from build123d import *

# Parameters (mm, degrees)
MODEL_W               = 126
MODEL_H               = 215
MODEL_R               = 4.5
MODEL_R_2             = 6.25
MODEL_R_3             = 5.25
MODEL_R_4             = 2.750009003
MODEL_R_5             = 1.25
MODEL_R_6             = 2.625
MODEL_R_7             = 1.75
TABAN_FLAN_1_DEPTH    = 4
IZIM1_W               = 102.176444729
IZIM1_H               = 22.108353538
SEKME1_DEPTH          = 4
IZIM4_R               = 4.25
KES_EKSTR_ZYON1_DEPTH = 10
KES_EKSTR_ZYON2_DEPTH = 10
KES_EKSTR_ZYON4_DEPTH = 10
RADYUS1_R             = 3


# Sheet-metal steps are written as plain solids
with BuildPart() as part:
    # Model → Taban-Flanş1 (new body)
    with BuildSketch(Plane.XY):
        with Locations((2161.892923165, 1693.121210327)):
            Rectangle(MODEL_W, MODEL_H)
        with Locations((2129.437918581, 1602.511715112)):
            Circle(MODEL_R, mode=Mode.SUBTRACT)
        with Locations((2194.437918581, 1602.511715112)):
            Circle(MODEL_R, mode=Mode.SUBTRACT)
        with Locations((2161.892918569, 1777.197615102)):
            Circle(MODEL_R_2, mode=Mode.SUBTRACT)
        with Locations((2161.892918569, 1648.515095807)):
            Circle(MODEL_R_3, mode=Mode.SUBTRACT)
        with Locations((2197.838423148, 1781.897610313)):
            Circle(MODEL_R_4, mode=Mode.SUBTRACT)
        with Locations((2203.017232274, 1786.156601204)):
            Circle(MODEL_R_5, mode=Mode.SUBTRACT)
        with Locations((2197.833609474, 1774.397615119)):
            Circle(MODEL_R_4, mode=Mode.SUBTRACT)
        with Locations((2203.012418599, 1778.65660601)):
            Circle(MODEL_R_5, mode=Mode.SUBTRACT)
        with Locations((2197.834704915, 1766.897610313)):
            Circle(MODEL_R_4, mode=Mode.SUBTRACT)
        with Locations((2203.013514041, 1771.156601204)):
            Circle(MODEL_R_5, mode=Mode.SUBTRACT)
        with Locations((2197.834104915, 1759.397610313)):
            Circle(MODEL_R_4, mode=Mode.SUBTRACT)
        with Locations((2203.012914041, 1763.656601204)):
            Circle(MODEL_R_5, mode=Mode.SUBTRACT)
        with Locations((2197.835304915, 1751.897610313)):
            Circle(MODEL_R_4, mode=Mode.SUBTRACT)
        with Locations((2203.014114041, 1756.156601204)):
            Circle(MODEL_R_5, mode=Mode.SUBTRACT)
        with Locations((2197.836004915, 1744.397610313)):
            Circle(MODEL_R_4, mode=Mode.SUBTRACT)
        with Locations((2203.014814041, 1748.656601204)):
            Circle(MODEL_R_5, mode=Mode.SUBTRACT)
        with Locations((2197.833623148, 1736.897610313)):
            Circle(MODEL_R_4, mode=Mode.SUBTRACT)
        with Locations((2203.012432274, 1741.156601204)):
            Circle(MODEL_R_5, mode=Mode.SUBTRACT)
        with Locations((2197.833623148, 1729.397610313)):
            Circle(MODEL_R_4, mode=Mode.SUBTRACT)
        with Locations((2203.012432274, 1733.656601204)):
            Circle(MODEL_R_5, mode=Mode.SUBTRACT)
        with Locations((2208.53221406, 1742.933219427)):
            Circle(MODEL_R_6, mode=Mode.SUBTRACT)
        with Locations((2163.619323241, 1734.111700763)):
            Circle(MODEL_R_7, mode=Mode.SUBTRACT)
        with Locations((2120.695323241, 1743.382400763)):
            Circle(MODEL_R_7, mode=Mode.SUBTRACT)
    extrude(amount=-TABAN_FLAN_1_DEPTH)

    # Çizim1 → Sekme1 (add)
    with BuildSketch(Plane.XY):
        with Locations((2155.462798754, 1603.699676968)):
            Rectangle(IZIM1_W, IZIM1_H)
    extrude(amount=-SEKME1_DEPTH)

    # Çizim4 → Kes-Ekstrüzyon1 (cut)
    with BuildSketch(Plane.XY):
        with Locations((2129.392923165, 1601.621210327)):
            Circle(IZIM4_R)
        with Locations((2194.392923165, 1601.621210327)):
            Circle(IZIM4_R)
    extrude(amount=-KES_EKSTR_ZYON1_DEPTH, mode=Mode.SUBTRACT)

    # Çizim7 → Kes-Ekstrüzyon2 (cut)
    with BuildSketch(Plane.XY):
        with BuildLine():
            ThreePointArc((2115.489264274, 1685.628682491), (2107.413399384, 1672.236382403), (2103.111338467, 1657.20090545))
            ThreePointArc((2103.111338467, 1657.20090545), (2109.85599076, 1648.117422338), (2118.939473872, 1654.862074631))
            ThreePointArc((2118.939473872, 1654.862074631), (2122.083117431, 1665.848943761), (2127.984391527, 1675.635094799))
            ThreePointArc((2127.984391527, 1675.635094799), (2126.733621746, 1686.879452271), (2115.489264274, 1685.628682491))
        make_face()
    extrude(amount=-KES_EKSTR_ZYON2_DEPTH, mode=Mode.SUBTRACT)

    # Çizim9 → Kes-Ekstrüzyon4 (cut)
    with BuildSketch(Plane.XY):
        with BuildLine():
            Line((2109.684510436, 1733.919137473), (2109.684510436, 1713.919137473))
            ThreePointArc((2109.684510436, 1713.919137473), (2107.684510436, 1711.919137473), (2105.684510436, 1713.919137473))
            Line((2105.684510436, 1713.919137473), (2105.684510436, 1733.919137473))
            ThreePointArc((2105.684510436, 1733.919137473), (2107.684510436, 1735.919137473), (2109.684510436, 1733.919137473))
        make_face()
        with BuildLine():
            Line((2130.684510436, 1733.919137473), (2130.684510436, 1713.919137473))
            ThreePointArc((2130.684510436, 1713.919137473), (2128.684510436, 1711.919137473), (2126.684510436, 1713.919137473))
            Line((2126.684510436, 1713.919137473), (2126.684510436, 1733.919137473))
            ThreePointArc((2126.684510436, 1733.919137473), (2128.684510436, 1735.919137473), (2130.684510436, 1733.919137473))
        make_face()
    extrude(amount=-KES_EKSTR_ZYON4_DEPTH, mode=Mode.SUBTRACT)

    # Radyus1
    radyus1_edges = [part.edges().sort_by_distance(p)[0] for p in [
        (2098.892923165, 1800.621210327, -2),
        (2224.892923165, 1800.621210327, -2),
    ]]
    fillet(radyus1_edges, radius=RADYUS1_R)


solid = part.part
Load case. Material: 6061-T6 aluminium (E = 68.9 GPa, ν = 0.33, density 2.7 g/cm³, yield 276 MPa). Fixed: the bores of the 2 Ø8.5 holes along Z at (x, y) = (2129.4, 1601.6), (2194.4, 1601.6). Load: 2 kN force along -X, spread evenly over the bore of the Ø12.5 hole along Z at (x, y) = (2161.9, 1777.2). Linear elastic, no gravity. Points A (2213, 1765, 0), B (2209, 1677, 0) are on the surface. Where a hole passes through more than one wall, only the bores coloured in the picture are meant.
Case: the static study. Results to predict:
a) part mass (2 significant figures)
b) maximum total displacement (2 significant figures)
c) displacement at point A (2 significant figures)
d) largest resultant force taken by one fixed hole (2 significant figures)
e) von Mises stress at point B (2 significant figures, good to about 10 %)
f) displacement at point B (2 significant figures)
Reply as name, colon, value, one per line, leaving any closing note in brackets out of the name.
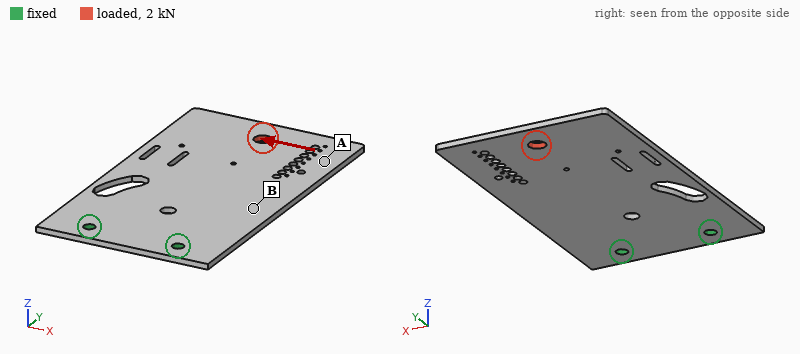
part mass: 280 g
maximum total displacement: 0.23 mm
displacement at point A: 0.18 mm
largest resultant force taken by one fixed hole: 5.1 kN
von Mises stress at point B: 16 MPa
displacement at point B: 0.073 mm
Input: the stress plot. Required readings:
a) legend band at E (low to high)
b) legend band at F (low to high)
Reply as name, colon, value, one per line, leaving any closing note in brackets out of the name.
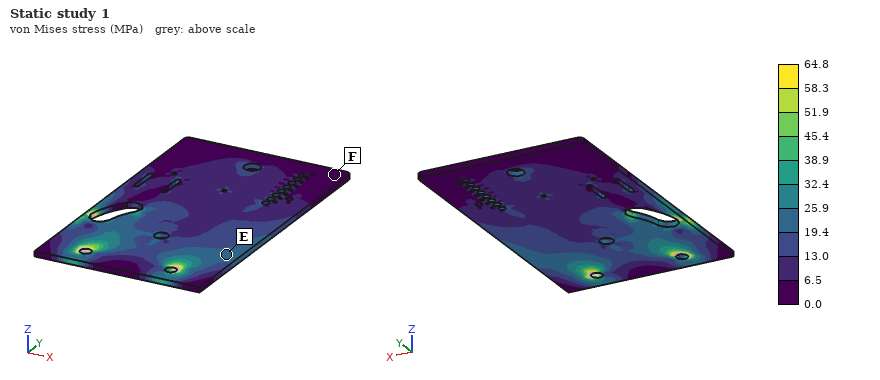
legend band at E: 19.4 to 25.9 MPa
legend band at F: 0.0 to 6.5 MPa
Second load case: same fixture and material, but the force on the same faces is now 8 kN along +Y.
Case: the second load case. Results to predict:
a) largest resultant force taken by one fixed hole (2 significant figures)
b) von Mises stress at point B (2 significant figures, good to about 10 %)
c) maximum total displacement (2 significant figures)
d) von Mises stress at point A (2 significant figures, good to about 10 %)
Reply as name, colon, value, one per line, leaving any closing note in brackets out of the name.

largest resultant force taken by one fixed hole: 4.0 kN
von Mises stress at point B: 13 MPa
maximum total displacement: 79 µm
von Mises stress at point A: 5.0 MPa
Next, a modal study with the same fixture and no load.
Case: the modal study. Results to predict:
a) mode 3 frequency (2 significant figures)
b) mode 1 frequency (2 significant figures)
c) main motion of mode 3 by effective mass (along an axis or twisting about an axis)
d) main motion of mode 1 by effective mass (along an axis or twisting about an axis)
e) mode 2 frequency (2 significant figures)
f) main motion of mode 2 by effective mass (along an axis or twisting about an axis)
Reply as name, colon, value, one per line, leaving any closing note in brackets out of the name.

mode 3 frequency: 520 Hz
mode 1 frequency: 82 Hz
main motion of mode 3 by effective mass: along Z
main motion of mode 1 by effective mass: along Z
mode 2 frequency: 280 Hz
main motion of mode 2 by effective mass: twisting about Y
